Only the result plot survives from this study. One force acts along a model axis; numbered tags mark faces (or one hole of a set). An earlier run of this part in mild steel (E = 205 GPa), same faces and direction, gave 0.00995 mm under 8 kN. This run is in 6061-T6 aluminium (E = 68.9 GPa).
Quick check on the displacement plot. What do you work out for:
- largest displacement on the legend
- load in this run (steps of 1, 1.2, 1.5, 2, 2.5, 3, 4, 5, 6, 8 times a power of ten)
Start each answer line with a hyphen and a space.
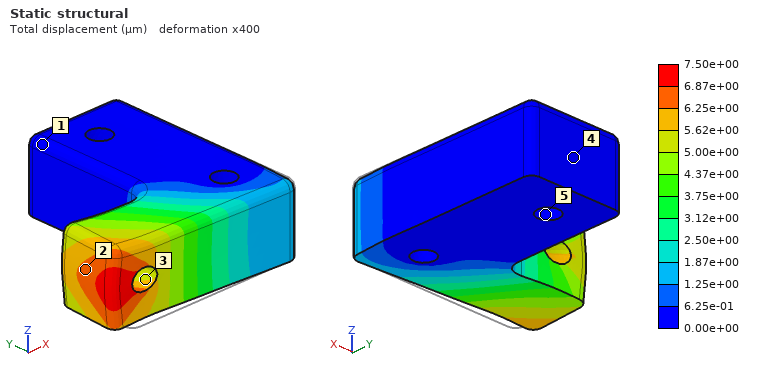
- 7.50e+00 µm
- 2 kN
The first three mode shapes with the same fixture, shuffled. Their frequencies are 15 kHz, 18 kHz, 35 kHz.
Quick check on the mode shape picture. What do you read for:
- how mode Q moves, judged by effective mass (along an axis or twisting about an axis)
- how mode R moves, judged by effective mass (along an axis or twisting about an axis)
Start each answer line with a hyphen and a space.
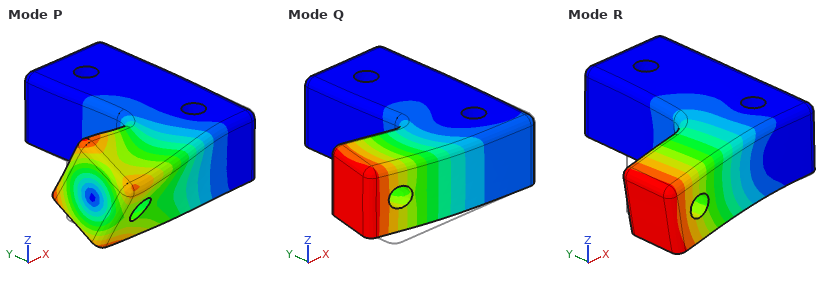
- along Y
- along Z
